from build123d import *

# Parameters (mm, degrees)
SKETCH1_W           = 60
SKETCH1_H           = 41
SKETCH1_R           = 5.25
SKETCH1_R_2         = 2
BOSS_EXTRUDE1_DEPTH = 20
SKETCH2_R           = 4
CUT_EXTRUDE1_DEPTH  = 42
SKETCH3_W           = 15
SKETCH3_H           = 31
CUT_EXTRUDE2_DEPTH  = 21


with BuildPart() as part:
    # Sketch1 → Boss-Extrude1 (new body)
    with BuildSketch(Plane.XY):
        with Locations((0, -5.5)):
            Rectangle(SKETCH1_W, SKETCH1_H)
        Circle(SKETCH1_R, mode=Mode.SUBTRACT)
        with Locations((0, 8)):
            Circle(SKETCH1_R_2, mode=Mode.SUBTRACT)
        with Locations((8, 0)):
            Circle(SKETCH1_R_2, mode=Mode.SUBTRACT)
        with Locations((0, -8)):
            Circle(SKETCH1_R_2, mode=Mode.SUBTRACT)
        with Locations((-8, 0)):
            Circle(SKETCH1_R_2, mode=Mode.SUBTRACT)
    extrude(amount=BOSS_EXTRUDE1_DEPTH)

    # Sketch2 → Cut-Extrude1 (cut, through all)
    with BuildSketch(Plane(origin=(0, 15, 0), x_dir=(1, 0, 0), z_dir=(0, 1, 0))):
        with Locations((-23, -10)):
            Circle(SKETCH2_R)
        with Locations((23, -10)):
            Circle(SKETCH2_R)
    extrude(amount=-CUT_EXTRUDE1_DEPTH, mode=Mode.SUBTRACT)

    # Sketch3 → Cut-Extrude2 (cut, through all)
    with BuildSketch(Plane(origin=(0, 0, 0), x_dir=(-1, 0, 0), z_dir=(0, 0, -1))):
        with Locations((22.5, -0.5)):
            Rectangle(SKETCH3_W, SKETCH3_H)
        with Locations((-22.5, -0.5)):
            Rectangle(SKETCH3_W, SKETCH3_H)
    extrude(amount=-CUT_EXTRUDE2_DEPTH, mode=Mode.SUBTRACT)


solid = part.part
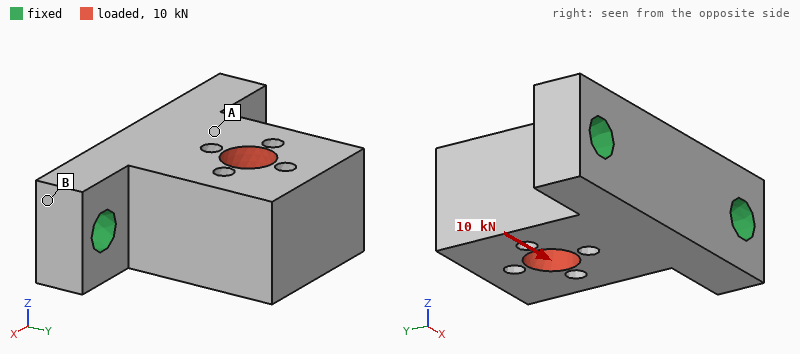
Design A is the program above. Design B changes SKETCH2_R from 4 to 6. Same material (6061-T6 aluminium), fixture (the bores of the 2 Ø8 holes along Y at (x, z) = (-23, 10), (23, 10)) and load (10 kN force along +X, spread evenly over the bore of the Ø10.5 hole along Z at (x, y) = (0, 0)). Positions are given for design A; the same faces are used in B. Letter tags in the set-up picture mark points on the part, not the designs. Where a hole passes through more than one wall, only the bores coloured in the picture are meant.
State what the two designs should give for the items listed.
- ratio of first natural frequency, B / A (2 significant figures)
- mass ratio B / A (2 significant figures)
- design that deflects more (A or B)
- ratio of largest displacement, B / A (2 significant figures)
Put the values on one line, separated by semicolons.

1.2; 0.95; A; 0.88
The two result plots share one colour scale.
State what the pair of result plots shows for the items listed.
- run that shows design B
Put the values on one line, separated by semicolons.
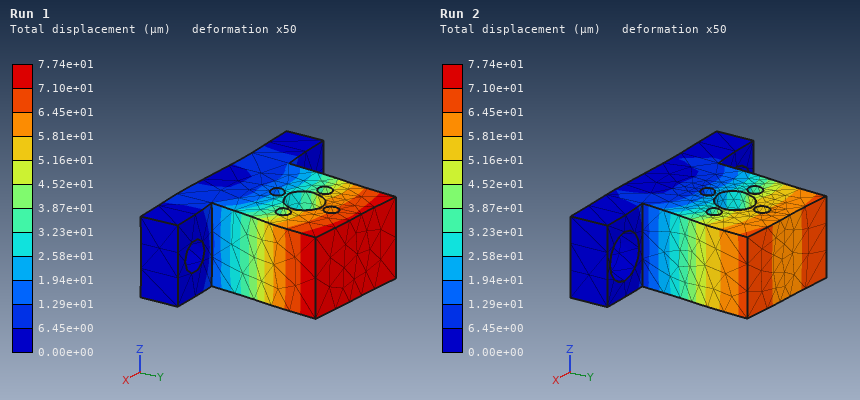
Run 2
